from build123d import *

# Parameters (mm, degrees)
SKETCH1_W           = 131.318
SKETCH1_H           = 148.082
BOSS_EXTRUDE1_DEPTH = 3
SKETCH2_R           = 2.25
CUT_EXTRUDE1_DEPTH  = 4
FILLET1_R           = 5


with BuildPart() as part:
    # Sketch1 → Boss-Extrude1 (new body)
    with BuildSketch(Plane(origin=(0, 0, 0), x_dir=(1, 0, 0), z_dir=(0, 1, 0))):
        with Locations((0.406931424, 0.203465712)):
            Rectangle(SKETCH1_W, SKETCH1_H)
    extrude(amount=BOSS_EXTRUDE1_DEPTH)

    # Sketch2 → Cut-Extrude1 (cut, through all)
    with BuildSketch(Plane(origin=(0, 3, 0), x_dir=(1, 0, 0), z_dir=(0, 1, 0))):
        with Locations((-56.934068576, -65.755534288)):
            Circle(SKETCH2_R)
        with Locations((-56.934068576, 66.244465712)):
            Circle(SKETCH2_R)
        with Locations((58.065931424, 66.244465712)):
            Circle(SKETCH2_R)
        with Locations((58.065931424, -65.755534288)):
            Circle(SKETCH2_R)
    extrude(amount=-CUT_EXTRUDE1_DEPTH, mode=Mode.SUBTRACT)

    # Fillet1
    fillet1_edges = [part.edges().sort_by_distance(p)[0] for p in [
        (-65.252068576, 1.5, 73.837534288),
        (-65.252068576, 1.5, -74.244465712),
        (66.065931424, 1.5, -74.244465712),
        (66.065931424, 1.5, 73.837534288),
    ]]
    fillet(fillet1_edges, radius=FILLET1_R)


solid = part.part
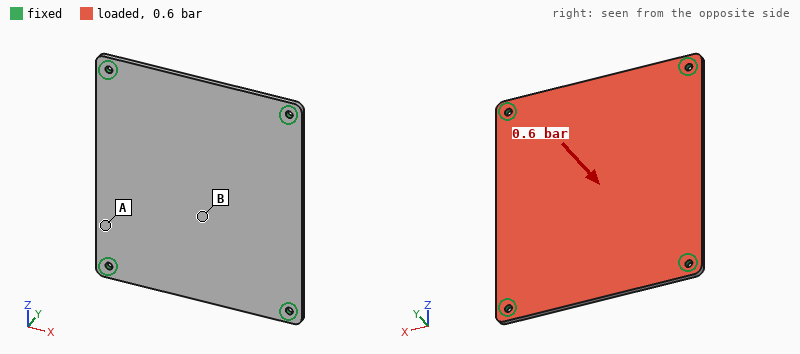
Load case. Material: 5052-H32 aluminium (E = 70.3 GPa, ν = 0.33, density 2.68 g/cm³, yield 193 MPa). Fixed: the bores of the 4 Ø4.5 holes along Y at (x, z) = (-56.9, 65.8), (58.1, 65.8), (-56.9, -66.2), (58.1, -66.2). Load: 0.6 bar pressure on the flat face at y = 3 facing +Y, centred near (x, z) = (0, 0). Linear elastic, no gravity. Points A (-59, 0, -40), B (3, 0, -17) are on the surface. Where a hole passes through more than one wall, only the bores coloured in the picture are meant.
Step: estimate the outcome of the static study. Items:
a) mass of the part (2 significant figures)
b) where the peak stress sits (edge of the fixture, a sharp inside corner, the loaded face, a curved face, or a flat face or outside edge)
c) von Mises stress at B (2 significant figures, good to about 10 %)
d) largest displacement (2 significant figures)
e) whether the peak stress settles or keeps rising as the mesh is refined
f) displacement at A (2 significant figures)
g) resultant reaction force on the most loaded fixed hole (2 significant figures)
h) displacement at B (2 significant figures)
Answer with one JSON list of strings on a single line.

["160 g", "edge of the fixture", "34 MPa", "0.68 mm", "keeps rising", "0.19 mm", "290 N", "0.64 mm"]
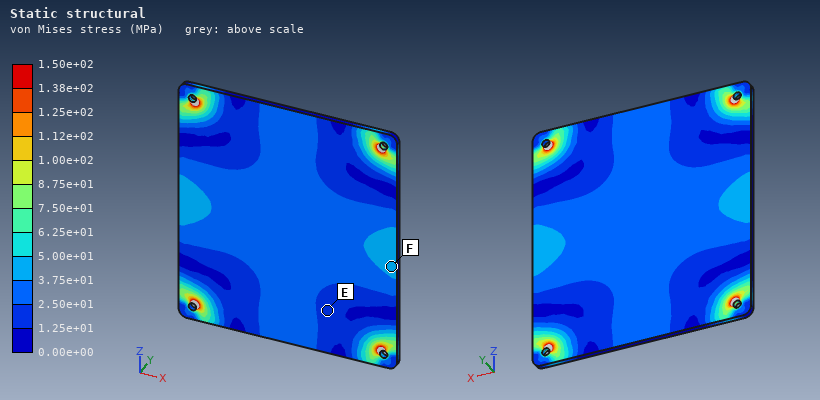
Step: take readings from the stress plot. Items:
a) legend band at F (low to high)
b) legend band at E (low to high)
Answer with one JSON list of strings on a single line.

["3.75e+01 to 5.00e+01 MPa", "1.25e+01 to 2.50e+01 MPa"]
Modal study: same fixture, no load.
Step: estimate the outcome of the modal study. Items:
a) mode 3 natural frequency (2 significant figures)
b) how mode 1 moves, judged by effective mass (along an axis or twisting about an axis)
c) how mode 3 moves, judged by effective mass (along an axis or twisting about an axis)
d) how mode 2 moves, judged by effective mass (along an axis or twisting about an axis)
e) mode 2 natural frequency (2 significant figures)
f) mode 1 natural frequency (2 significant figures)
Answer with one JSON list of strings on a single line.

["1200 Hz", "along Y", "twisting about X", "twisting about Z", "1000 Hz", "630 Hz"]
